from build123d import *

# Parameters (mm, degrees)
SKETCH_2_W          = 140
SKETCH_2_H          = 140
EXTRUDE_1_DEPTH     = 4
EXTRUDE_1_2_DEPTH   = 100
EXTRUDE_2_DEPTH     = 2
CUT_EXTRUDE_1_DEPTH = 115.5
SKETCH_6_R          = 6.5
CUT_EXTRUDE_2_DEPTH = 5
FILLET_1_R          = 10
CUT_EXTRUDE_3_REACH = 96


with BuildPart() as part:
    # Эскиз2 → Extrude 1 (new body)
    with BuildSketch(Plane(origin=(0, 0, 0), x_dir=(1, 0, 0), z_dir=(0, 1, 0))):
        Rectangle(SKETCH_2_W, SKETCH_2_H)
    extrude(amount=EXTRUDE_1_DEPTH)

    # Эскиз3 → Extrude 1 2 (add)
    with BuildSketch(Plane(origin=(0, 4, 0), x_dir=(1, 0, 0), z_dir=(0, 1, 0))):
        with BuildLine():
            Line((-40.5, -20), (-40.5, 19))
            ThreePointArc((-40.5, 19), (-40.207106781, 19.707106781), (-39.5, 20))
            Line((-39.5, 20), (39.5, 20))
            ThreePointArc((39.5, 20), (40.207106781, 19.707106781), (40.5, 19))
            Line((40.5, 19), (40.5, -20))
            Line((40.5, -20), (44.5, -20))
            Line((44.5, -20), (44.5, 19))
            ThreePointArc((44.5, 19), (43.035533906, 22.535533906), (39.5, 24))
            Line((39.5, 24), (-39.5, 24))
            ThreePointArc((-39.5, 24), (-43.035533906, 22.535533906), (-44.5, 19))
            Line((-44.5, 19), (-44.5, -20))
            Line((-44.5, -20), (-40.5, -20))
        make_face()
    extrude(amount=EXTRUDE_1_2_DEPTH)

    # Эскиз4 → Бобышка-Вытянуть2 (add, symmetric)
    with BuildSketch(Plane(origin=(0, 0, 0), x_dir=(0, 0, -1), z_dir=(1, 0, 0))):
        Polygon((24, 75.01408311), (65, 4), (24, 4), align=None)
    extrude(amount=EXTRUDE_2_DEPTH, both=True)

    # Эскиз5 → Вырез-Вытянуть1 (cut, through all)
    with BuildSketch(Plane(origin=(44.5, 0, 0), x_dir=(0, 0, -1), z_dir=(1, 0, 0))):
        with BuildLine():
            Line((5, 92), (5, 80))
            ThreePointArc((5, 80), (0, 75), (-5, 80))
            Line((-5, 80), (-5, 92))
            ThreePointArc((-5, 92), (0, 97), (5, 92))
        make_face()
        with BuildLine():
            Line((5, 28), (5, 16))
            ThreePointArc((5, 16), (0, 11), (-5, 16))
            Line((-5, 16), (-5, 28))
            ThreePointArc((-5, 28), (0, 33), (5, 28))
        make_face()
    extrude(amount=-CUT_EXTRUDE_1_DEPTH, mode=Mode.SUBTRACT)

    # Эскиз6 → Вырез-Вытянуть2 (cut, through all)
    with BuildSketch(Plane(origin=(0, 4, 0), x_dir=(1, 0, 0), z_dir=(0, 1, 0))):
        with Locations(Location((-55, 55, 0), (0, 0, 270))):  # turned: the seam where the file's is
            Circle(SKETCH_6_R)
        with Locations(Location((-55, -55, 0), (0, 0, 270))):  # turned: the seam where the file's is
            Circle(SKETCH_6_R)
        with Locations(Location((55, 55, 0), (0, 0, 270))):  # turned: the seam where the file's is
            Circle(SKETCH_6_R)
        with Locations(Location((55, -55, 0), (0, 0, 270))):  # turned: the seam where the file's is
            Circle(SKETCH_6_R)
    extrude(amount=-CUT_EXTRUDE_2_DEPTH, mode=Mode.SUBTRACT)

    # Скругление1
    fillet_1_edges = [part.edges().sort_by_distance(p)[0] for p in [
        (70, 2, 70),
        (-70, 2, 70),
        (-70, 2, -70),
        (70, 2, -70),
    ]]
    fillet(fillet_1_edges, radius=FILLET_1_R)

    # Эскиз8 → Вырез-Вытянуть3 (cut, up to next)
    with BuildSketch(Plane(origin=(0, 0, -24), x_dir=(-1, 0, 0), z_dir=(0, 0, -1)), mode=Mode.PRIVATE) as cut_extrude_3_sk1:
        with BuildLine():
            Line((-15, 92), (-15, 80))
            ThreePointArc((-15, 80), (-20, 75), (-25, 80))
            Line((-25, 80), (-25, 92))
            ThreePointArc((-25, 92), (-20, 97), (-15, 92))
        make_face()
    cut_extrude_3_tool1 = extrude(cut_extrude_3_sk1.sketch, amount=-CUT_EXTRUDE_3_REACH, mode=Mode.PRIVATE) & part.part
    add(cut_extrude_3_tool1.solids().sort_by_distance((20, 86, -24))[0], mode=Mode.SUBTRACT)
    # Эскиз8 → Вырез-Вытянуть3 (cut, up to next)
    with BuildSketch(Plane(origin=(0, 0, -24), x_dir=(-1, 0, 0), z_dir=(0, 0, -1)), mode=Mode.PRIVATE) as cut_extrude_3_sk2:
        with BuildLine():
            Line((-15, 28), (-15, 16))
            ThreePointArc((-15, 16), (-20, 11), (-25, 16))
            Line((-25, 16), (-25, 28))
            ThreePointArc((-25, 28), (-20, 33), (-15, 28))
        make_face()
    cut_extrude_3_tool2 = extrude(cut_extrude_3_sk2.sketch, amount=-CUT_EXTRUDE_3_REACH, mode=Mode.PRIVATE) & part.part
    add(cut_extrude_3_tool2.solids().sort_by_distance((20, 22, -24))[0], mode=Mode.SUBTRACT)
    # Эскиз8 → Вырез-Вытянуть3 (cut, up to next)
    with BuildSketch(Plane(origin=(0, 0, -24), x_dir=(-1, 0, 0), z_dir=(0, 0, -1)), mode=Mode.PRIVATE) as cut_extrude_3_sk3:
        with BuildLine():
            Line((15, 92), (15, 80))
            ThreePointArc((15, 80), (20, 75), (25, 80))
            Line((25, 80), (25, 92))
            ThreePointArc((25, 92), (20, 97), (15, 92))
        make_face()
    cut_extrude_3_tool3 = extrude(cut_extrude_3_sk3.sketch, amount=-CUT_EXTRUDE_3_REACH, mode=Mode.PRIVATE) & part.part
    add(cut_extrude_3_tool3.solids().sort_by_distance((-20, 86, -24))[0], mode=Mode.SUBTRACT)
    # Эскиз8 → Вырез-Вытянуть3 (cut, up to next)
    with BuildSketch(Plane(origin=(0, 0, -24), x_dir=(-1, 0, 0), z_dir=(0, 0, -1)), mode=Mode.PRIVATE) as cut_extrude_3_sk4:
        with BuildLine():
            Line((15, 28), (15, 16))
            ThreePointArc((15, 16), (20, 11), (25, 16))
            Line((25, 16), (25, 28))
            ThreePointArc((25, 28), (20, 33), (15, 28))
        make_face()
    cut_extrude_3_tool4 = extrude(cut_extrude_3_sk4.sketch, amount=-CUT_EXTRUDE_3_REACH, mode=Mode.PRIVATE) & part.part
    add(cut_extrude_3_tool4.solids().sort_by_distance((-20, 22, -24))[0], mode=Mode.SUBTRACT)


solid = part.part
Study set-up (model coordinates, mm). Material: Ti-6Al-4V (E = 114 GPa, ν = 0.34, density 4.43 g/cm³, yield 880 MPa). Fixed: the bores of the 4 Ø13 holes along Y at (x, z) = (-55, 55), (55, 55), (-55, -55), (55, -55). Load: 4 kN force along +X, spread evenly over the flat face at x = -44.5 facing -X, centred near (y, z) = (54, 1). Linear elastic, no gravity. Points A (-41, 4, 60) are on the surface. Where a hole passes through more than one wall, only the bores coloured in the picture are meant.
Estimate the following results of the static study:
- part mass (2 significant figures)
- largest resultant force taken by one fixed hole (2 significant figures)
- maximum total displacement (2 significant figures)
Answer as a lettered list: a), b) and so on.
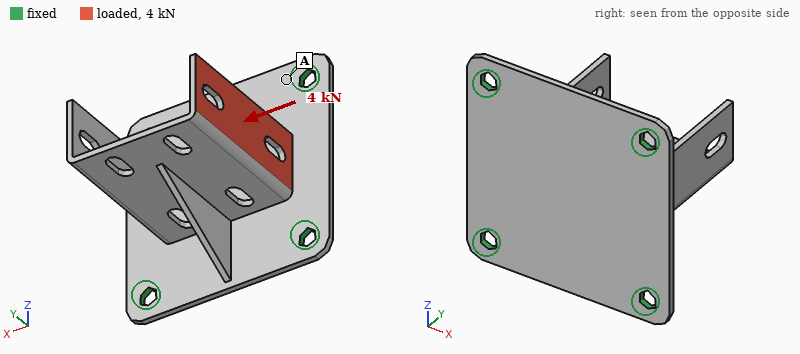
a) 630 g
b) 2.3 kN
c) 2.3 mm
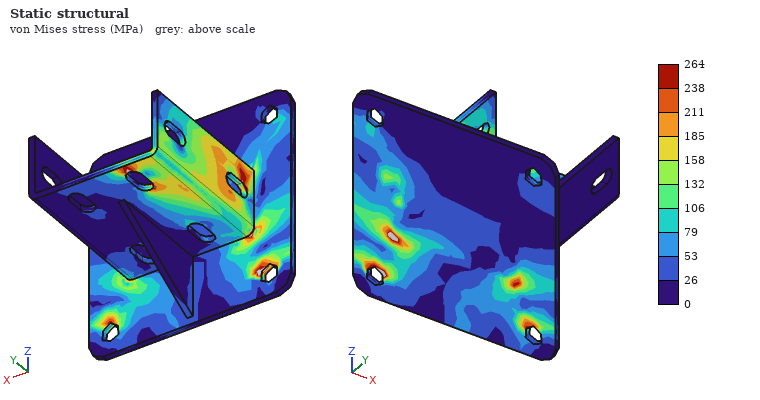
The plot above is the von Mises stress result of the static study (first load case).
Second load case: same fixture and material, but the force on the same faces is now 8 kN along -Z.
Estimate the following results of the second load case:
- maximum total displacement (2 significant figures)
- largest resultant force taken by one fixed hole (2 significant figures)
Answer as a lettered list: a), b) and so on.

a) 2.7 mm
b) 5.6 kN
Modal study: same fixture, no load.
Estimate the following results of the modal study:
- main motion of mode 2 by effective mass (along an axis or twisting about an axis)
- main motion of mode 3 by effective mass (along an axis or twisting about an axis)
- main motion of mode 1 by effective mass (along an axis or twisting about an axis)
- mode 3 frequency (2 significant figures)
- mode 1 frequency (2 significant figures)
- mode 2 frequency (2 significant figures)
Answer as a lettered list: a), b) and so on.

a) along Z
b) along Y
c) along X
d) 1200 Hz
e) 830 Hz
f) 940 Hz
